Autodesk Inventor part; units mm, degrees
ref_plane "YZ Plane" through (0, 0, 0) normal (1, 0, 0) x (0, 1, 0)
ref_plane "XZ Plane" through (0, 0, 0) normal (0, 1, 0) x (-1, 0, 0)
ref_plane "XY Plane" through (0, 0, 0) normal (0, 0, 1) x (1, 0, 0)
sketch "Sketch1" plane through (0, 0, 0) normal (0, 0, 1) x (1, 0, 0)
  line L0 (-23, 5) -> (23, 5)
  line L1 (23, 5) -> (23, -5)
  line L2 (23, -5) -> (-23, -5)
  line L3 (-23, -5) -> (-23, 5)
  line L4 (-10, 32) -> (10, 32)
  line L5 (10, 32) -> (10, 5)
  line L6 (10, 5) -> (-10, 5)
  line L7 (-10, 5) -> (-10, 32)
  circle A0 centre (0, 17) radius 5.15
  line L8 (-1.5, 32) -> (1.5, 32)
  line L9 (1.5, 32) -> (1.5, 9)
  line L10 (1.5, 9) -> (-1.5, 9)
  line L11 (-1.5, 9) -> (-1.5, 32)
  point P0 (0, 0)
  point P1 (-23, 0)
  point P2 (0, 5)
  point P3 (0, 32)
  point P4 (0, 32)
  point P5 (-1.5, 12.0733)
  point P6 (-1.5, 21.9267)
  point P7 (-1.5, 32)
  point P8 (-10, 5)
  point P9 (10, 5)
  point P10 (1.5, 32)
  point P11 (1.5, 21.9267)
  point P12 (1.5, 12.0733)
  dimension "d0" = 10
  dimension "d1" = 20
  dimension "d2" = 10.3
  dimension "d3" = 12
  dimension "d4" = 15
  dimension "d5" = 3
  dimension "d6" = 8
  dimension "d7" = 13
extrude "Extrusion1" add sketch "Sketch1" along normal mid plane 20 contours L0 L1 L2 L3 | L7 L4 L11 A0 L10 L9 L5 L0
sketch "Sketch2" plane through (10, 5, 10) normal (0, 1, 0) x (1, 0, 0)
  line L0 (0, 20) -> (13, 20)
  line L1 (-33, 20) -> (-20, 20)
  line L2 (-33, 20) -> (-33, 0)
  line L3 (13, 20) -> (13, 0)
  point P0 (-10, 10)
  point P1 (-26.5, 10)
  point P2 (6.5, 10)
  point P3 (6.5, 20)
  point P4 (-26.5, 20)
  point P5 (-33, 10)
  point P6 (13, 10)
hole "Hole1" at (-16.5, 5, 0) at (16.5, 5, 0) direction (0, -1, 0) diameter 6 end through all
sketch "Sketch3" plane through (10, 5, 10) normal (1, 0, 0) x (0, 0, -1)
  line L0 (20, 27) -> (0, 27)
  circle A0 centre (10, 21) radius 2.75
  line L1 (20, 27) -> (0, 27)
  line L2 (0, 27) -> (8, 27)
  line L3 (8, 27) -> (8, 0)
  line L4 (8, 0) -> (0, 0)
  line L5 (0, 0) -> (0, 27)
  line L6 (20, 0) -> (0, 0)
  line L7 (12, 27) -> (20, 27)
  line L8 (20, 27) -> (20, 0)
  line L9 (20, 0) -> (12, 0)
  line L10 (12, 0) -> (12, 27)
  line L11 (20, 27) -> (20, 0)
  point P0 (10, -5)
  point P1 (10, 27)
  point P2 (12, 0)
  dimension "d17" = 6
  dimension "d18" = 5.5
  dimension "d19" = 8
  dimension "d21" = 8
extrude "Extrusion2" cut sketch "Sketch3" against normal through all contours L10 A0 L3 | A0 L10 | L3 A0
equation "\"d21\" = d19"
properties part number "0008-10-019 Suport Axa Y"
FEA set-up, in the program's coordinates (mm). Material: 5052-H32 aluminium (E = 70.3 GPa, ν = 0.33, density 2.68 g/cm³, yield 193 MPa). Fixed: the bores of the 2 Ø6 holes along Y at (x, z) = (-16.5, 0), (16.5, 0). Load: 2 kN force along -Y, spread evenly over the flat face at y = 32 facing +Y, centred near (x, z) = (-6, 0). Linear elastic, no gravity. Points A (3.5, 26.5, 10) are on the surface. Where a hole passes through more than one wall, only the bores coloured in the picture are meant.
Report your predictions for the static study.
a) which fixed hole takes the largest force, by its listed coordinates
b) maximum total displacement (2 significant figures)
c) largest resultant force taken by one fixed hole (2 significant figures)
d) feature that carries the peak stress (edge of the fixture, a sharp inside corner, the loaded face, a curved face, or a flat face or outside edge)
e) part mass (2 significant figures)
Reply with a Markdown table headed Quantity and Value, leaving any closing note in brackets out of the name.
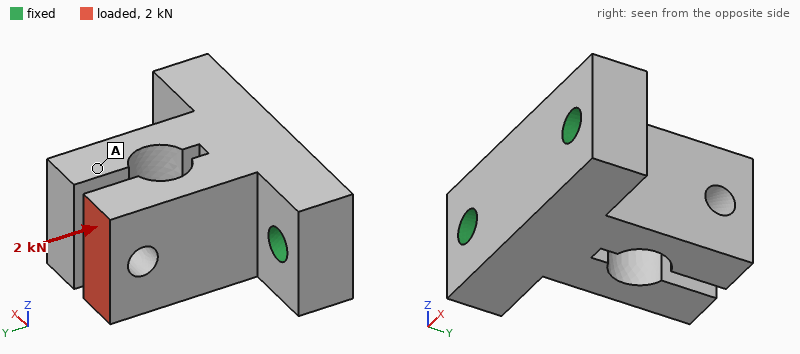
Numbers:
| Quantity | Value |
|---|---|
| which fixed hole takes the largest force, by its listed coordinates | (-16.5, 0) |
| maximum total displacement | 35 µm |
| largest resultant force taken by one fixed hole | 1.5 kN |
| feature that carries the peak stress | a curved face |
| part mass | 44 g |
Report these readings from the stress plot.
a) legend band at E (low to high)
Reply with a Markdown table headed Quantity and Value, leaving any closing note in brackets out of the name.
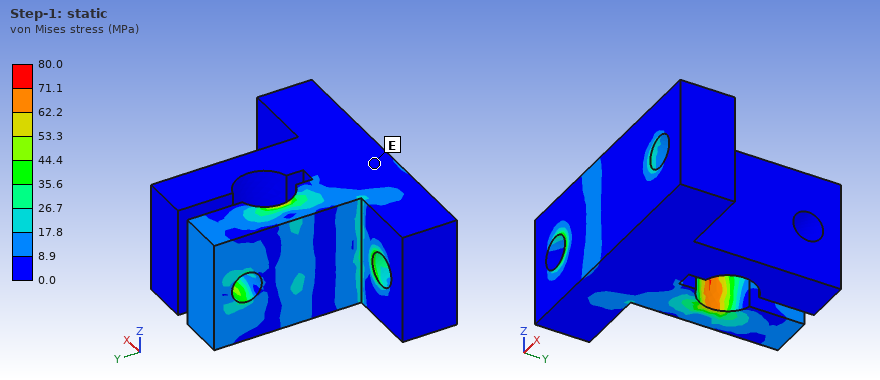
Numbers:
| Quantity | Value |
|---|---|
| legend band at E | 0.0 to 8.9 MPa |
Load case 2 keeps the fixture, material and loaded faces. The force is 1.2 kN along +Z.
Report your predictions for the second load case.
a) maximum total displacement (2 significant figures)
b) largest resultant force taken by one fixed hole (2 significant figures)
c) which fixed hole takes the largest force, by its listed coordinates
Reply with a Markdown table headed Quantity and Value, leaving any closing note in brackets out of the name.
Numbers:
| Quantity | Value |
|---|---|
| maximum total displacement | 99 µm |
| largest resultant force taken by one fixed hole | 800 N |
| which fixed hole takes the largest force, by its listed coordinates | (-16.5, 0) |
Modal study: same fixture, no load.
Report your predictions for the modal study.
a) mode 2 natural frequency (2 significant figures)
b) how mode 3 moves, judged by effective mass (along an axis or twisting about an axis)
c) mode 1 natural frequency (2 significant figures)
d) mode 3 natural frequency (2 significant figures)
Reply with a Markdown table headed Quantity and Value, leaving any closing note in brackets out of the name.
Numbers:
| Quantity | Value |
|---|---|
| mode 2 natural frequency | 7000 Hz |
| how mode 3 moves, judged by effective mass | along Z |
| mode 1 natural frequency | 7000 Hz |
| mode 3 natural frequency | 7700 Hz |
